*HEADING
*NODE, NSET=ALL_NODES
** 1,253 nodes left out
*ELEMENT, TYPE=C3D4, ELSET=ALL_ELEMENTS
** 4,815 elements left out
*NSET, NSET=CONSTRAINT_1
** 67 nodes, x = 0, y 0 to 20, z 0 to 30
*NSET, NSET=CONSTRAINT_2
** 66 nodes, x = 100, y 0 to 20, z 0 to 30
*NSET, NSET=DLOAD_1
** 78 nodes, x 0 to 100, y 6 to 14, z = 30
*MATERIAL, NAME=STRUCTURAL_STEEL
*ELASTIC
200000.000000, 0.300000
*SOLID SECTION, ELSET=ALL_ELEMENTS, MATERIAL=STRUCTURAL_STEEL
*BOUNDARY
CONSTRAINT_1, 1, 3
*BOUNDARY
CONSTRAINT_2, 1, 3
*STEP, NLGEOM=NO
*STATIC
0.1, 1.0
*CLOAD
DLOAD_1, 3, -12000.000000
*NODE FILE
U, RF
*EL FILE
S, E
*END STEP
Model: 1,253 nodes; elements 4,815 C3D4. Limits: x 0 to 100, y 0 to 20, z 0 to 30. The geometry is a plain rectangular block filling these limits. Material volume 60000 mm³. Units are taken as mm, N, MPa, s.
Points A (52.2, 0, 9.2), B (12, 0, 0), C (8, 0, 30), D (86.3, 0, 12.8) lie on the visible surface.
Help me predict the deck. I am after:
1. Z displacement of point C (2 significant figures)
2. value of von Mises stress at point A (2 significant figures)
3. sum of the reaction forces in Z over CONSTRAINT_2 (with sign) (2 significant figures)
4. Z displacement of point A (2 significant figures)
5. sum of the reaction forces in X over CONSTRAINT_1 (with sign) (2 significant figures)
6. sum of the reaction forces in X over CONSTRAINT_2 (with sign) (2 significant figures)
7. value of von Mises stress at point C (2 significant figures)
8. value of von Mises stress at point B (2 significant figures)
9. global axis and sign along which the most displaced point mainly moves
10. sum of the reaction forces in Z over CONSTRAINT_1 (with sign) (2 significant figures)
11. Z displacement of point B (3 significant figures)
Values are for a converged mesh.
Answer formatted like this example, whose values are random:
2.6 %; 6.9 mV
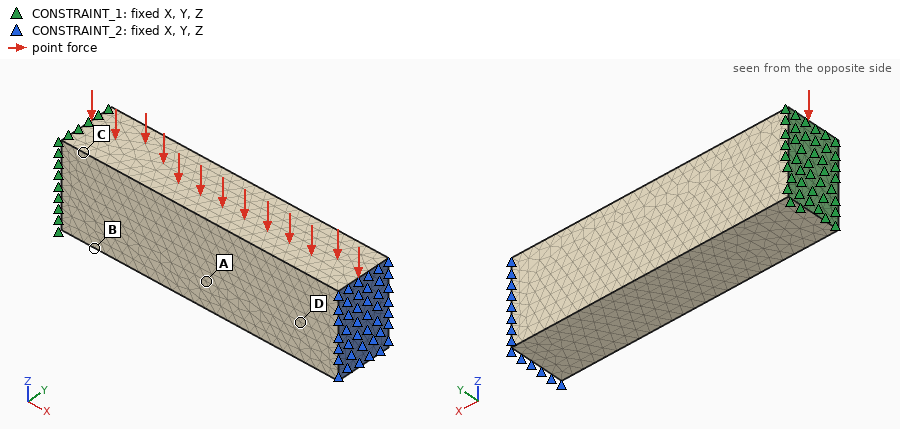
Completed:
-0.10 mm; 450 MPa; 4.7e+05 N; -0.53 mm; 38000 N; -38000 N; 1300 MPa; 850 MPa; -Z; 4.6e+05 N; -0.155 mm
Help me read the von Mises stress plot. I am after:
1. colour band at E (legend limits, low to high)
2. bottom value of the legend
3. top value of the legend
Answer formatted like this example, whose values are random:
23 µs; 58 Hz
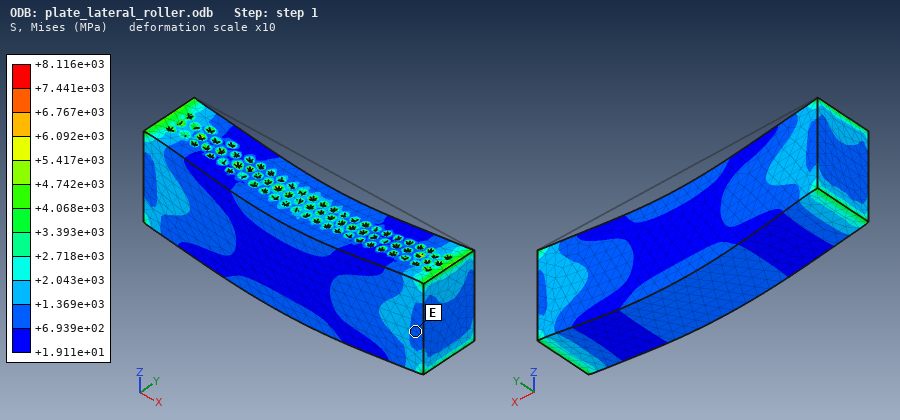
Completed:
+6.939e+02 to +1.369e+03 MPa; +1.911e+01 MPa; +8.116e+03 MPa
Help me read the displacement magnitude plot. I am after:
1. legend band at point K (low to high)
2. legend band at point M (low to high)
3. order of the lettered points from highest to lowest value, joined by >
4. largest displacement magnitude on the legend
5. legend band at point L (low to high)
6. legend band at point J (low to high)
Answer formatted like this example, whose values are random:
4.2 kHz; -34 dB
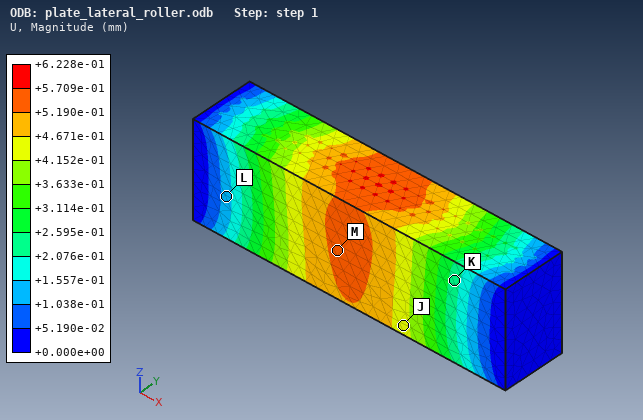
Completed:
+2.076e-01 to +2.595e-01 mm; +5.190e-01 to +5.709e-01 mm; M > J > K > L; +6.228e-01 mm; +1.038e-01 to +1.557e-01 mm; +4.152e-01 to +4.671e-01 mm
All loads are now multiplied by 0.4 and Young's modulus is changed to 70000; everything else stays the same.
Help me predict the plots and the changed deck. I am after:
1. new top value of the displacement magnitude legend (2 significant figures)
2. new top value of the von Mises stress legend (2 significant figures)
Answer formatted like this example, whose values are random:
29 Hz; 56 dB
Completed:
0.71 mm; 3200 MPa
